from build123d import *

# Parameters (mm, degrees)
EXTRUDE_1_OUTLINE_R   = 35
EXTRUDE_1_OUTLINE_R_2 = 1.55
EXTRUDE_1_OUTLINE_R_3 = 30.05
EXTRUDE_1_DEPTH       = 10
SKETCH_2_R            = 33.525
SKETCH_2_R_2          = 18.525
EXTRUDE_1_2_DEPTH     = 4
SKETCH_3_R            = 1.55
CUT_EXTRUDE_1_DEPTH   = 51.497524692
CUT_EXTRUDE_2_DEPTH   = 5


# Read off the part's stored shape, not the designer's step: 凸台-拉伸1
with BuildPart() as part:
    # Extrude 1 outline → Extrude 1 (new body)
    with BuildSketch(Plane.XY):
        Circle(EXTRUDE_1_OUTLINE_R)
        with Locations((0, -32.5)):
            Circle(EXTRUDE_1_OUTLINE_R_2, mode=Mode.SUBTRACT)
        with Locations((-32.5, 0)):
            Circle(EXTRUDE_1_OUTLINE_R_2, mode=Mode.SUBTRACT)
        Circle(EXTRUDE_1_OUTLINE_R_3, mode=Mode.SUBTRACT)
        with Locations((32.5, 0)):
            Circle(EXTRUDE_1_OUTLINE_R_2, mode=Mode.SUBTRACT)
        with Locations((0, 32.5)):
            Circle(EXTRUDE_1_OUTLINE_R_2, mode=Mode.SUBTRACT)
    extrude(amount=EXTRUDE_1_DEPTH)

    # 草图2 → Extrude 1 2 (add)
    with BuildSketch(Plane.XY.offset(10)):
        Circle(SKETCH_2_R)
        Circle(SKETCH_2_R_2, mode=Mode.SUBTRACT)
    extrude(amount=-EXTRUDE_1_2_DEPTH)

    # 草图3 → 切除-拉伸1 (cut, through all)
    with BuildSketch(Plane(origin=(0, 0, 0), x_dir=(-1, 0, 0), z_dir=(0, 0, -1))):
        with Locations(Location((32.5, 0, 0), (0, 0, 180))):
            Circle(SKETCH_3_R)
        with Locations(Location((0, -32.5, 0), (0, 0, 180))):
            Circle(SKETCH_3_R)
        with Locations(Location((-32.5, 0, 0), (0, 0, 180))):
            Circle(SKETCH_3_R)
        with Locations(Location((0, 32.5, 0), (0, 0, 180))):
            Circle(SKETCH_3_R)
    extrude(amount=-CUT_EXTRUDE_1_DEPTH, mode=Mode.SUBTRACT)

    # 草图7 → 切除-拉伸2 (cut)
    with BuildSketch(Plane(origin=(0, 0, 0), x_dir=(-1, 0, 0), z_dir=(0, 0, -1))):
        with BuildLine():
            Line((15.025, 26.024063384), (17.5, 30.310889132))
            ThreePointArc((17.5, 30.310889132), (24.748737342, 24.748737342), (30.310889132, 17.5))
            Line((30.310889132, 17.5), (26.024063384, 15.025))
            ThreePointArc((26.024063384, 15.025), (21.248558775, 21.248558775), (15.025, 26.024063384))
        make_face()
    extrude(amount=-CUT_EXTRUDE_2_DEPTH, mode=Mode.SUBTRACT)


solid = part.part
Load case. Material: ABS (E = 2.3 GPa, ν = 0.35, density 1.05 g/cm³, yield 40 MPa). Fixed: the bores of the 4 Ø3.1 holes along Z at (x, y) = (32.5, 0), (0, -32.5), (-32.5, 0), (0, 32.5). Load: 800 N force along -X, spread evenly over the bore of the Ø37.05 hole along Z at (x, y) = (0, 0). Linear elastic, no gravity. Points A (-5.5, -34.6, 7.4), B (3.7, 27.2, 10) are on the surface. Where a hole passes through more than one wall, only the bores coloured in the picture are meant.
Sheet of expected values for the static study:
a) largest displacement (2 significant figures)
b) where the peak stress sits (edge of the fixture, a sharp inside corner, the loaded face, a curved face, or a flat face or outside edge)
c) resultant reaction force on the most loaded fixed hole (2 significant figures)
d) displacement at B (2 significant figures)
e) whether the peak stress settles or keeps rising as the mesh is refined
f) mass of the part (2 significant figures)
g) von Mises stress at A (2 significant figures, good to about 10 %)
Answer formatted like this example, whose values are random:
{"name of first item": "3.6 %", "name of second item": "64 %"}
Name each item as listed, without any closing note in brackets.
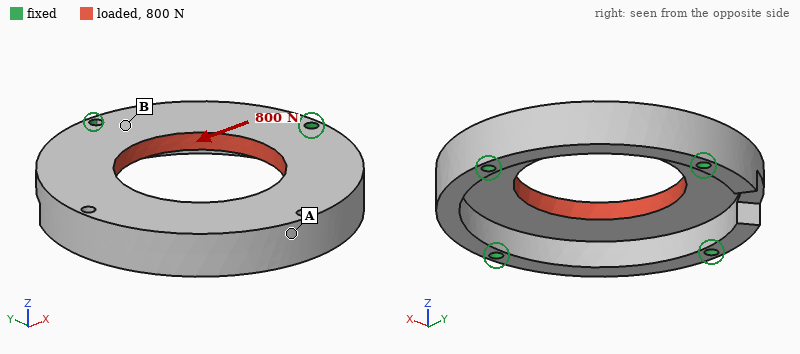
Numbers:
{"largest displacement": "56 µm", "where the peak stress sits": "edge of the fixture", "resultant reaction force on the most loaded fixed hole": "210 N", "displacement at B": "24 µm", "whether the peak stress settles or keeps rising as the mesh is refined": "keeps rising", "mass of the part": "17 g", "von Mises stress at A": "2.5 MPa"}
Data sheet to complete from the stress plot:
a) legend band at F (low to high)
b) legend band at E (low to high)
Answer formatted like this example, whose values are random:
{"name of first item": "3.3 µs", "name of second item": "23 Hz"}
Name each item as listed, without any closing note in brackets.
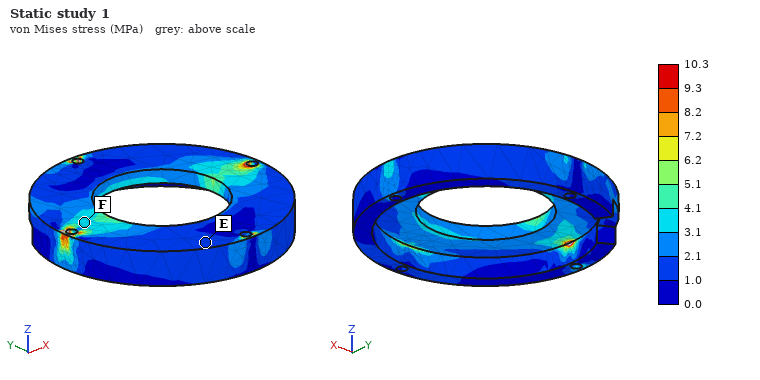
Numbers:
{"legend band at F": "3.1 to 4.1 MPa", "legend band at E": "1.0 to 2.1 MPa"}
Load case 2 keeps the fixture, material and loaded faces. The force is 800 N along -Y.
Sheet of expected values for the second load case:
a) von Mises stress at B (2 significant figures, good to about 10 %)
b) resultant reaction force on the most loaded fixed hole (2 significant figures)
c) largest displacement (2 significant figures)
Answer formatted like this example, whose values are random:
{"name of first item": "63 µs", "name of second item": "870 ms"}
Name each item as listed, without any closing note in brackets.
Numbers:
{"von Mises stress at B": "3.8 MPa", "resultant reaction force on the most loaded fixed hole": "240 N", "largest displacement": "60 µm"}
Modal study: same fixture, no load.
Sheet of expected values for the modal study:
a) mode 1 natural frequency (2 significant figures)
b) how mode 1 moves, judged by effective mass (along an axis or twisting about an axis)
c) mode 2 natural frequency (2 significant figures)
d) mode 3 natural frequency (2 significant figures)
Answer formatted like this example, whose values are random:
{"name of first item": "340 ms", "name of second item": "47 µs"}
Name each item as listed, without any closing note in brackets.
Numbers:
{"mode 1 natural frequency": "3600 Hz", "how mode 1 moves, judged by effective mass": "along Z", "mode 2 natural frequency": "3900 Hz", "mode 3 natural frequency": "4100 Hz"}
